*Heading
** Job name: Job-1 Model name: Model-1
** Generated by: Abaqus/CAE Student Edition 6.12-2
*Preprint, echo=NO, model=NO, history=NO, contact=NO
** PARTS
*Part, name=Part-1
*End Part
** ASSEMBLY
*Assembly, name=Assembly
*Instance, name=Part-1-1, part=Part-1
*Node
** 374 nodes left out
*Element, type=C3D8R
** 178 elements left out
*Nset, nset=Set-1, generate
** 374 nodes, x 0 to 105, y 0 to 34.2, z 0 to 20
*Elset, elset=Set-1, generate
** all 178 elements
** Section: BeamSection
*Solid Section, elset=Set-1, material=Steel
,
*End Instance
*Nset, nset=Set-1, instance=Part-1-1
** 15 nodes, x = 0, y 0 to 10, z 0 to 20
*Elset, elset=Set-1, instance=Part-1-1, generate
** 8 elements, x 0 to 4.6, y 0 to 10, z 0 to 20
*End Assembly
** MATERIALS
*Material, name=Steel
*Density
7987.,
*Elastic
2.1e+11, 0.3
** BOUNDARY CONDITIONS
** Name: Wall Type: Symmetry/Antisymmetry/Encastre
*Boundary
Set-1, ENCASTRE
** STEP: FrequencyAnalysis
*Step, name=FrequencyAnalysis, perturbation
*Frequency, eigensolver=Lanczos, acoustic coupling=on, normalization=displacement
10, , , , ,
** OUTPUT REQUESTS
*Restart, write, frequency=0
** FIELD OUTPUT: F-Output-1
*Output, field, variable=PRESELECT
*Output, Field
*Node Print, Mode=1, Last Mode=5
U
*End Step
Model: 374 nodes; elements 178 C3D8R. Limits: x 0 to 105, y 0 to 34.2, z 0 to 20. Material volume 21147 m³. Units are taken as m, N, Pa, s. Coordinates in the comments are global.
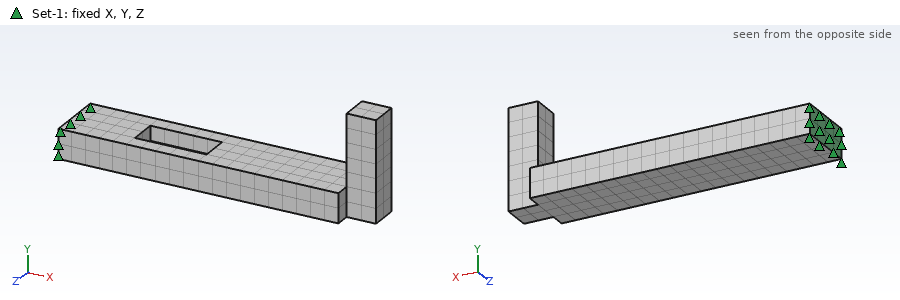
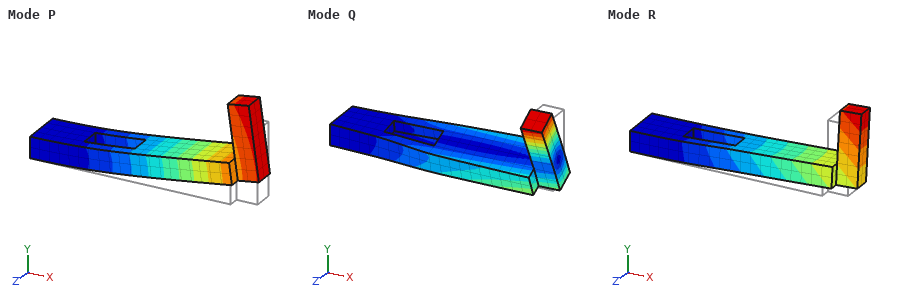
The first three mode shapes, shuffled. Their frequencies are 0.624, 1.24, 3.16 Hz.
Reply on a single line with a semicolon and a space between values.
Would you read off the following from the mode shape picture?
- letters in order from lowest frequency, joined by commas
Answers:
P, R, Q
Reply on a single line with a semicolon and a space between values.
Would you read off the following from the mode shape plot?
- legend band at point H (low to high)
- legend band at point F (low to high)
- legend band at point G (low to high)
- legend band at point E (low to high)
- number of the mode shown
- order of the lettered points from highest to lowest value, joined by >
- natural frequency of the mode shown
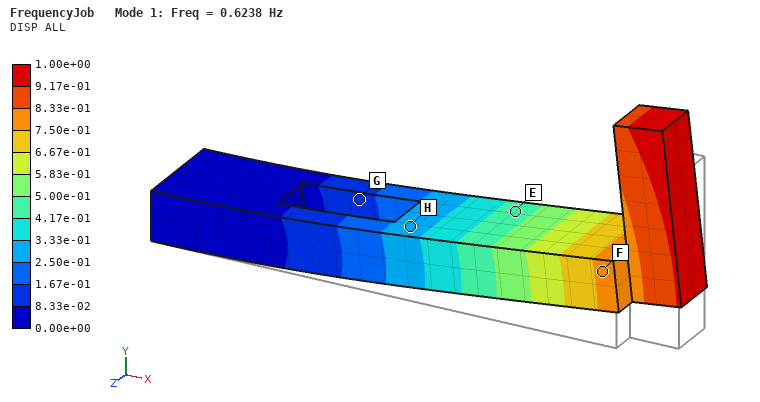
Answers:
2.50e-01 to 3.33e-01; 7.50e-01 to 8.33e-01; 8.33e-02 to 1.67e-01; 4.17e-01 to 5.00e-01; 1; F > E > H > G; 0.6238 Hz
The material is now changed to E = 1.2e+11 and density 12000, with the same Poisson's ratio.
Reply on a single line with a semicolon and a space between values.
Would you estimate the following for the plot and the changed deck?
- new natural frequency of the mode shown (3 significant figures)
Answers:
0.385 Hz
